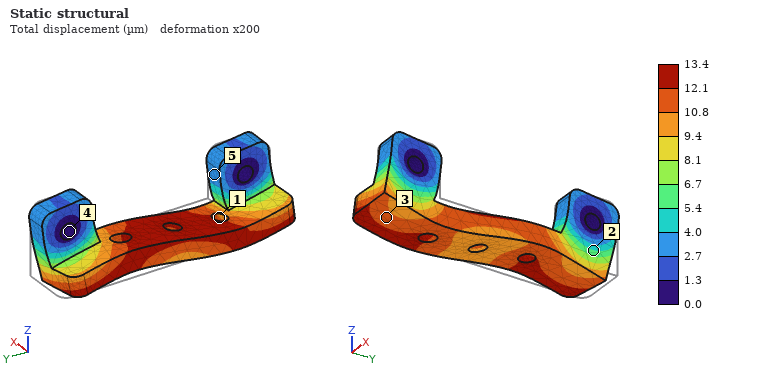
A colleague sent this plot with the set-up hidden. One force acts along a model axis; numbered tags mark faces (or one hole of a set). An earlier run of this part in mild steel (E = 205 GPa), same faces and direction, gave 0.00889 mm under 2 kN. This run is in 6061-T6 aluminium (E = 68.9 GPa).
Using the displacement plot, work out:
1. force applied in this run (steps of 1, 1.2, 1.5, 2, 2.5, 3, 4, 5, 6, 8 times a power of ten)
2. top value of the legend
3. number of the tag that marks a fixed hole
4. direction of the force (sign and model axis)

1 kN
13.4 µm
4
-Y
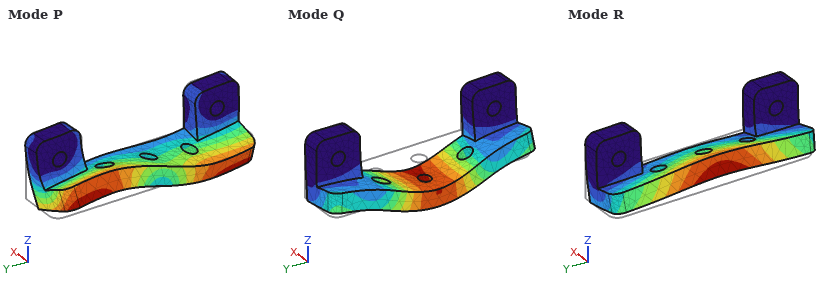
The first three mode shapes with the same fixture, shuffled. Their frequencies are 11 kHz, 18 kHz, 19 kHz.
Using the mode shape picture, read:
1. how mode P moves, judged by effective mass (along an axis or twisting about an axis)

along Y
